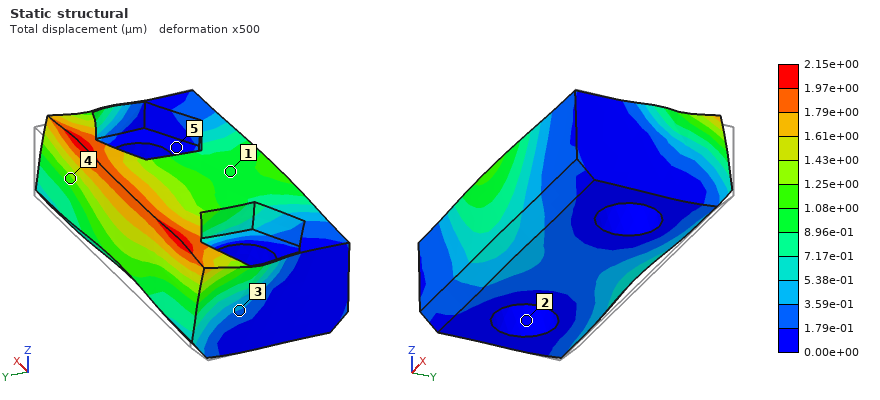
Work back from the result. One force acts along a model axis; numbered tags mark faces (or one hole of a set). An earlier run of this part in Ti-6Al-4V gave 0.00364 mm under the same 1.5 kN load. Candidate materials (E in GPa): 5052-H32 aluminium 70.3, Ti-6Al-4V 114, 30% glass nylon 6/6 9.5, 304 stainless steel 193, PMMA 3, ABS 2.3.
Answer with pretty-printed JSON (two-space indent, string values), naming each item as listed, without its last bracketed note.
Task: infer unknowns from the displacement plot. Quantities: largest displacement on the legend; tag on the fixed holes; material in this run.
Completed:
{
  "largest displacement on the legend": "2.15e+00 µm",
  "tag on the fixed holes": "2",
  "material in this run": "304 stainless steel"
}
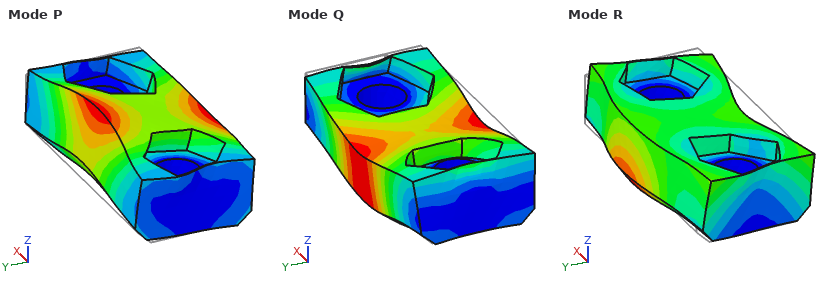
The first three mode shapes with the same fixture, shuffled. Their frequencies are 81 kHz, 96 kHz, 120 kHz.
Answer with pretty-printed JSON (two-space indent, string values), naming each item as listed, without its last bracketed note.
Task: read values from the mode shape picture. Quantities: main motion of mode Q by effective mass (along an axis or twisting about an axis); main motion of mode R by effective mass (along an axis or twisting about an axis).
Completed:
{
  "main motion of mode Q by effective mass": "along Z",
  "main motion of mode R by effective mass": "along Y"
}
